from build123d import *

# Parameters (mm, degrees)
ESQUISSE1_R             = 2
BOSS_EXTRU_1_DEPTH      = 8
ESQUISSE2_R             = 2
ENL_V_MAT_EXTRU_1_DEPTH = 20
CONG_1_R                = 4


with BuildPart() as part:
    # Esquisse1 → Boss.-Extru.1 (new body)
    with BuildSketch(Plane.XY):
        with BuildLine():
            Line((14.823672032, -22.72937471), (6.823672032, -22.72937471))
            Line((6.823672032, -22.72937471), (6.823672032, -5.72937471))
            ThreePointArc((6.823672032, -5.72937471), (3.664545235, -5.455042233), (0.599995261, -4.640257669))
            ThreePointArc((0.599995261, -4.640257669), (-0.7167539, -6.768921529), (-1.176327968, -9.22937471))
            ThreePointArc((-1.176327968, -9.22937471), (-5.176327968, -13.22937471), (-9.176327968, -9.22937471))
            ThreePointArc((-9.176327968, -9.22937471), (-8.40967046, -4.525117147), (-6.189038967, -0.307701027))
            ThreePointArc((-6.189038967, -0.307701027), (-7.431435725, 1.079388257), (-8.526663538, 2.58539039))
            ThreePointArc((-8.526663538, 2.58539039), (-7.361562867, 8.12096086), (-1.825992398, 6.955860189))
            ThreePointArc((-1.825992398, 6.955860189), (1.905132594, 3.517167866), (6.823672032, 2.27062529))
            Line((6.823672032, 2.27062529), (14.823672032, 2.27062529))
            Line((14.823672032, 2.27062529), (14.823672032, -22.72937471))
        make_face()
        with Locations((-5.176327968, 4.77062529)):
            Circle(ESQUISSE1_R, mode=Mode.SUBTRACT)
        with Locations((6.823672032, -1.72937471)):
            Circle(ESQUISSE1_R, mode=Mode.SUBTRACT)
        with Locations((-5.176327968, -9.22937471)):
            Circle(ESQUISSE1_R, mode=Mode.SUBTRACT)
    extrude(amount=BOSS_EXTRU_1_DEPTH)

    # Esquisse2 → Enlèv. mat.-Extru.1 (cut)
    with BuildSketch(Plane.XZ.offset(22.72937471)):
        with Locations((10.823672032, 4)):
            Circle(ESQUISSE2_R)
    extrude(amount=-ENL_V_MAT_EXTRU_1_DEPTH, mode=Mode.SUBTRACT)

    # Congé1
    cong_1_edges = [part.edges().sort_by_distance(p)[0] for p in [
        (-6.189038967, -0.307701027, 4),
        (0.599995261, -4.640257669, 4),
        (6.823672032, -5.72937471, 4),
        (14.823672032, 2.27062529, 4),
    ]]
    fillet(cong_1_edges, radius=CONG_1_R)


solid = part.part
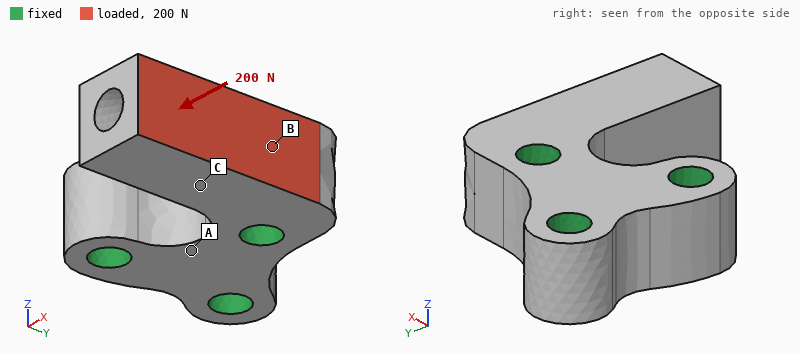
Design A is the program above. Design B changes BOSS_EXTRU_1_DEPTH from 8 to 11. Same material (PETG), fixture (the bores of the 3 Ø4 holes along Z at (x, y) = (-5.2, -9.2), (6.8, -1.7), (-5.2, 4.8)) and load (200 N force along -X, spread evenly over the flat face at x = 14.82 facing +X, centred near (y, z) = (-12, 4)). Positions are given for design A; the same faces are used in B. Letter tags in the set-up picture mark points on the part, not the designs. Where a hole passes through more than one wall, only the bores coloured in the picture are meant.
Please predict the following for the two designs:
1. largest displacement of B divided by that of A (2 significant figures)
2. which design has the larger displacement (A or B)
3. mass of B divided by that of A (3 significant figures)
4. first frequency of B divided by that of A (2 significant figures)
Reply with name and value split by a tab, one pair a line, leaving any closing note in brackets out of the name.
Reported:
largest displacement of B divided by that of A	0.70
which design has the larger displacement	A
mass of B divided by that of A	1.41
first frequency of B divided by that of A	0.99
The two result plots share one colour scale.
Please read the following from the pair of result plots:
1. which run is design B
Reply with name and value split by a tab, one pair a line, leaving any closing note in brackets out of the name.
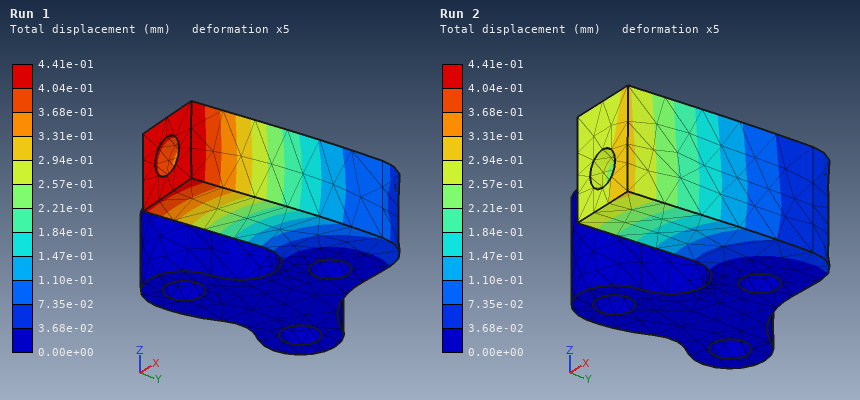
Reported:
which run is design B	Run 2
